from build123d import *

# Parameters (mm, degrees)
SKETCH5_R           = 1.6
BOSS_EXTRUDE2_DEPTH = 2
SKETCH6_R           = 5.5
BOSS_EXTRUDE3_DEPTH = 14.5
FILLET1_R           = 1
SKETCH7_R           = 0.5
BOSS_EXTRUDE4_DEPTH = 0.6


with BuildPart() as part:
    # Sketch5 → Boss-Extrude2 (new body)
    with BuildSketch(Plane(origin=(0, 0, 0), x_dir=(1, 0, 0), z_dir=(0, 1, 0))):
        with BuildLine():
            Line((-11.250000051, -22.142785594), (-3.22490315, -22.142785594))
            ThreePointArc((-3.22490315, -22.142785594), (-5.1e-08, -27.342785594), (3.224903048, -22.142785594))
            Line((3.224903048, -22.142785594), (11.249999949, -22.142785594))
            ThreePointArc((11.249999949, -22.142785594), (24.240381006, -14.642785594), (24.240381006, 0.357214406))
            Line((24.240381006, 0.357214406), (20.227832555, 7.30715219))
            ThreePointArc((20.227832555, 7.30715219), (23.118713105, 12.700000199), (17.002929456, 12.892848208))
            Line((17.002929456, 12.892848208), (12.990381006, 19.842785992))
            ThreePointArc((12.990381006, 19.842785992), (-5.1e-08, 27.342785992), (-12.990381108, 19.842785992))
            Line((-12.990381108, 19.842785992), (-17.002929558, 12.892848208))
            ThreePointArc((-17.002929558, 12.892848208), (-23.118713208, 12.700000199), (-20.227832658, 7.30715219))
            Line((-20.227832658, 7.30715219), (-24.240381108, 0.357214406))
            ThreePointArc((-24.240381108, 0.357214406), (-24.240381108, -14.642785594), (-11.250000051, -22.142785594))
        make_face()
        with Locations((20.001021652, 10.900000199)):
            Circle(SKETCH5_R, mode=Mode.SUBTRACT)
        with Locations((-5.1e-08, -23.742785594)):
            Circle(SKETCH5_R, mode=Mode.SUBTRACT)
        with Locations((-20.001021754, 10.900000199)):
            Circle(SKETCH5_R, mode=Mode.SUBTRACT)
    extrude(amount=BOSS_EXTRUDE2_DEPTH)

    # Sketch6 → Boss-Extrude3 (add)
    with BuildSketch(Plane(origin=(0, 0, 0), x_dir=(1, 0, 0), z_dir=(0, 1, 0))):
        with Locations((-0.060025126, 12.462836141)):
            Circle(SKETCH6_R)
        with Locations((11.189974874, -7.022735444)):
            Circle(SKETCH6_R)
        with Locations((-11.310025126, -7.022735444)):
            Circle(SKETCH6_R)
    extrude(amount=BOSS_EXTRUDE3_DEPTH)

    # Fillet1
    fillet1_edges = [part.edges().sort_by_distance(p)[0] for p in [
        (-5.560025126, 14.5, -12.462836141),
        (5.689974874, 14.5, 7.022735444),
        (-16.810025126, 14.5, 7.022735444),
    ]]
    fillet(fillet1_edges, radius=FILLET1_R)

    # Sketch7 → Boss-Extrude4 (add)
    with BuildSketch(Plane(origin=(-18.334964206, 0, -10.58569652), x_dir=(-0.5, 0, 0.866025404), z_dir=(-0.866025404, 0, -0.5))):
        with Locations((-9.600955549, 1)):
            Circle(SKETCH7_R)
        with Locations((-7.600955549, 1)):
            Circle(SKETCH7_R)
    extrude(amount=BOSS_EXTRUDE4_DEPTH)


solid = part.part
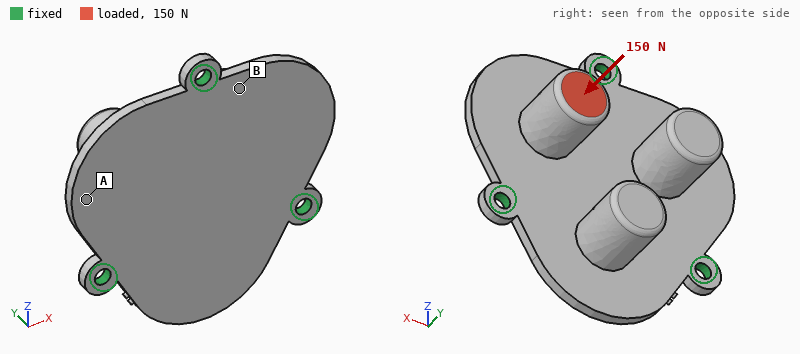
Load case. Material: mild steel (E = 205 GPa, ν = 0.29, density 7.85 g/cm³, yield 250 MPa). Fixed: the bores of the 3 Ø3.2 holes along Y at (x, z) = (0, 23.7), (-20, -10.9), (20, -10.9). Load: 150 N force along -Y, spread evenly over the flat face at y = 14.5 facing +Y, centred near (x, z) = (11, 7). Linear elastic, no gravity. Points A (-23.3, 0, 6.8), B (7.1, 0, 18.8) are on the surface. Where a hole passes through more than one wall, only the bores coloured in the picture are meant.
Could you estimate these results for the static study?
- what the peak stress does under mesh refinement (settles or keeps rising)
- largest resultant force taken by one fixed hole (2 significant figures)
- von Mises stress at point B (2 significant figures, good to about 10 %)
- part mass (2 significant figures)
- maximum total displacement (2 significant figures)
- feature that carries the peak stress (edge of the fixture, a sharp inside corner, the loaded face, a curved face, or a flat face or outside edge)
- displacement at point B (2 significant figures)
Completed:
keeps rising
78 N
14 MPa
59 g
24 µm
edge of the fixture
8.2 µm
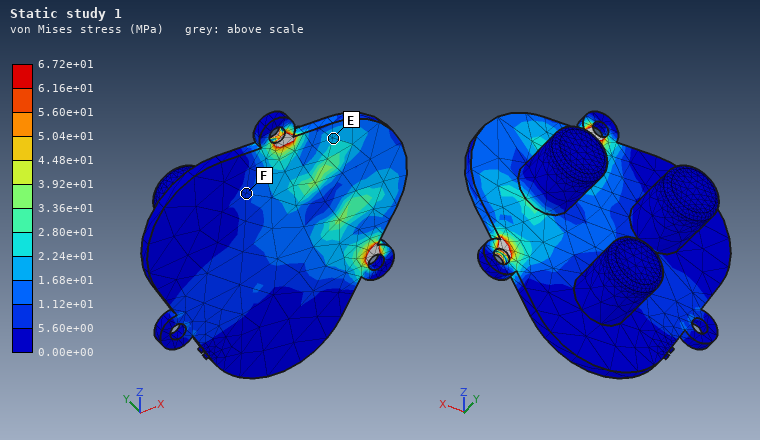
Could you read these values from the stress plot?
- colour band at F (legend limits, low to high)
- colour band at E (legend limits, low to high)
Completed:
5.60e+00 to 1.12e+01 MPa
1.68e+01 to 2.24e+01 MPa
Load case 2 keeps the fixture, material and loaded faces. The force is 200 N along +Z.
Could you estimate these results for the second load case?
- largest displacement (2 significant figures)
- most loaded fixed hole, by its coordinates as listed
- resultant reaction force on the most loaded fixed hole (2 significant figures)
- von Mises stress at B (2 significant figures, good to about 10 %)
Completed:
33 µm
(0, 23.7)
130 N
28 MPa
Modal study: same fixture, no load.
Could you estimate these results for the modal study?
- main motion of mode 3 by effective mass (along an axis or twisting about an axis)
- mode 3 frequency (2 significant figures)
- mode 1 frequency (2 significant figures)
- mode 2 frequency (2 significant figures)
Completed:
along Y
3800 Hz
3200 Hz
3200 Hz
